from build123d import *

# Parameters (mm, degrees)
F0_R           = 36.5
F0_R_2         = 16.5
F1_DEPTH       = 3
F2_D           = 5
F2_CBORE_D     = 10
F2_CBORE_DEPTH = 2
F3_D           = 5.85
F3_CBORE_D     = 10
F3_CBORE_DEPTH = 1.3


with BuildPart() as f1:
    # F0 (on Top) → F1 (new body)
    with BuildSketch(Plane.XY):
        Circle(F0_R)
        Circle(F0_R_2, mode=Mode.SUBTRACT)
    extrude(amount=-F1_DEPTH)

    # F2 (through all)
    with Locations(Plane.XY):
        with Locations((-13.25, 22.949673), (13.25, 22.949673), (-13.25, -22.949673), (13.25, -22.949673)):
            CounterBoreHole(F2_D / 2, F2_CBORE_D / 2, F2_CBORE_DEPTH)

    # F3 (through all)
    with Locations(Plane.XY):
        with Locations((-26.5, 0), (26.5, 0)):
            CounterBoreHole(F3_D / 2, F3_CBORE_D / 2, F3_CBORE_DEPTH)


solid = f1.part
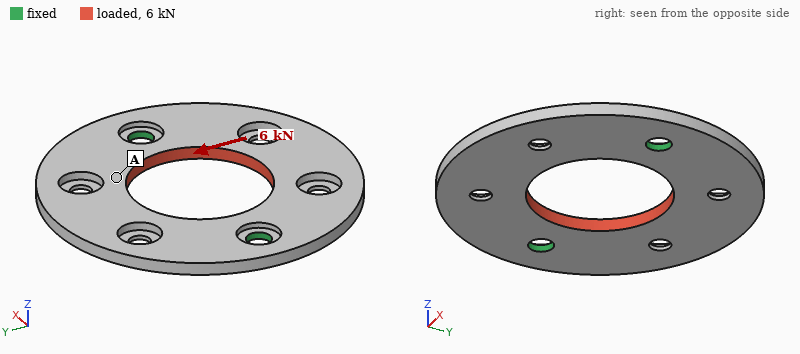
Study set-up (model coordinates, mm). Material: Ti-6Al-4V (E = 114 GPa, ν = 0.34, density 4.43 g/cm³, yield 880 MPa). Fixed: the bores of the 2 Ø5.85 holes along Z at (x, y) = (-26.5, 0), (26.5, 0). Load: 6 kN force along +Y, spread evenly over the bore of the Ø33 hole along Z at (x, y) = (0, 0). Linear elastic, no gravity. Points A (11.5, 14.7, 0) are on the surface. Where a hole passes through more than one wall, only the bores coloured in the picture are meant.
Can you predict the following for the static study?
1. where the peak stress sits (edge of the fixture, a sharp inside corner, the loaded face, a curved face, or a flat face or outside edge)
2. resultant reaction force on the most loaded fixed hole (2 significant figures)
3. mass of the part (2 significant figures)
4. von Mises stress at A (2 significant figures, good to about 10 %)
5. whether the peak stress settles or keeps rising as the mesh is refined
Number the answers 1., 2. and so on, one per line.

1. edge of the fixture
2. 3.0 kN
3. 40 g
4. 38 MPa
5. keeps rising
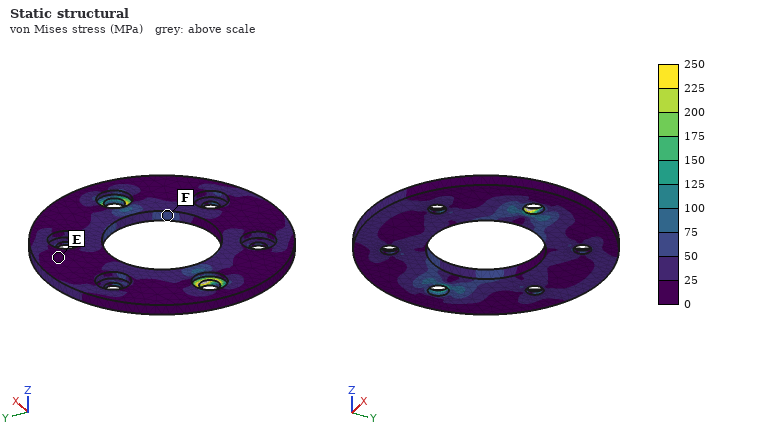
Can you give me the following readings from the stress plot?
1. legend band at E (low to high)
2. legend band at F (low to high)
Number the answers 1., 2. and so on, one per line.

1. 0 to 25 MPa
2. 50 to 75 MPa
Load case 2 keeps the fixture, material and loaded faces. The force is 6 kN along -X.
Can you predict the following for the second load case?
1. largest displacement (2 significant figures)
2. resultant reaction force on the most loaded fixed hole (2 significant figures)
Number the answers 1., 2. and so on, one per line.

1. 17 µm
2. 3.0 kN
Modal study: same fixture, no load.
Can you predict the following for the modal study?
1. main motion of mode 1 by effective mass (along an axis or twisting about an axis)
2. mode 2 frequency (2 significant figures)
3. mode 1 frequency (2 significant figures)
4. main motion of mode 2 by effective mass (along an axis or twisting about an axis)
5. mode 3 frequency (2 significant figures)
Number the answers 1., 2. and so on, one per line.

1. twisting about X
2. 1700 Hz
3. 1500 Hz
4. along Z
5. 3900 Hz
